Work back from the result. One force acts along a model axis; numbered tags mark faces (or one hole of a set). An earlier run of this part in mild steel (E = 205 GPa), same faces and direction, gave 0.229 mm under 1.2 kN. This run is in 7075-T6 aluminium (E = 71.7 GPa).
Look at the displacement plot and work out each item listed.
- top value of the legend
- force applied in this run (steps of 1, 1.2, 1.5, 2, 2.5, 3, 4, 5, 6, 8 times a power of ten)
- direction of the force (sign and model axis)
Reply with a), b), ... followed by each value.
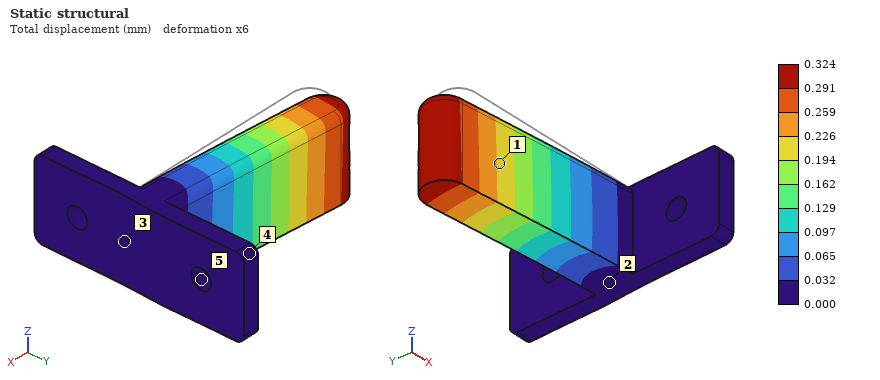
a) 0.324 mm
b) 600 N
c) +Y
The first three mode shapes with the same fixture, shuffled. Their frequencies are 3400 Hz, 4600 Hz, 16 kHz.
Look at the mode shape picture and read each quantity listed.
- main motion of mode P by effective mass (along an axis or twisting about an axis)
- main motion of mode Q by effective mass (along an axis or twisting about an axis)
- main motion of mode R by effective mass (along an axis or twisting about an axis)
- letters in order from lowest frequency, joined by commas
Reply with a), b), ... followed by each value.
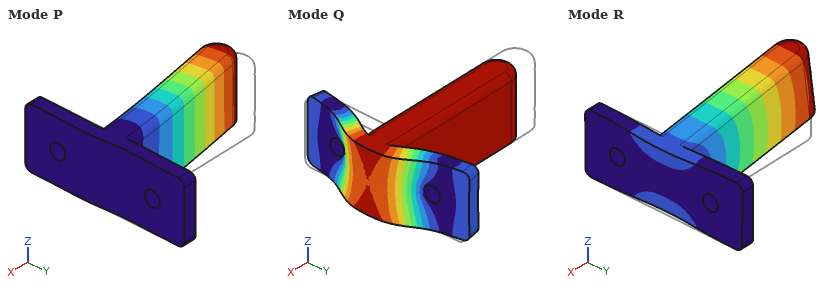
a) along Y
b) along X
c) along Z
d) R, P, Q
